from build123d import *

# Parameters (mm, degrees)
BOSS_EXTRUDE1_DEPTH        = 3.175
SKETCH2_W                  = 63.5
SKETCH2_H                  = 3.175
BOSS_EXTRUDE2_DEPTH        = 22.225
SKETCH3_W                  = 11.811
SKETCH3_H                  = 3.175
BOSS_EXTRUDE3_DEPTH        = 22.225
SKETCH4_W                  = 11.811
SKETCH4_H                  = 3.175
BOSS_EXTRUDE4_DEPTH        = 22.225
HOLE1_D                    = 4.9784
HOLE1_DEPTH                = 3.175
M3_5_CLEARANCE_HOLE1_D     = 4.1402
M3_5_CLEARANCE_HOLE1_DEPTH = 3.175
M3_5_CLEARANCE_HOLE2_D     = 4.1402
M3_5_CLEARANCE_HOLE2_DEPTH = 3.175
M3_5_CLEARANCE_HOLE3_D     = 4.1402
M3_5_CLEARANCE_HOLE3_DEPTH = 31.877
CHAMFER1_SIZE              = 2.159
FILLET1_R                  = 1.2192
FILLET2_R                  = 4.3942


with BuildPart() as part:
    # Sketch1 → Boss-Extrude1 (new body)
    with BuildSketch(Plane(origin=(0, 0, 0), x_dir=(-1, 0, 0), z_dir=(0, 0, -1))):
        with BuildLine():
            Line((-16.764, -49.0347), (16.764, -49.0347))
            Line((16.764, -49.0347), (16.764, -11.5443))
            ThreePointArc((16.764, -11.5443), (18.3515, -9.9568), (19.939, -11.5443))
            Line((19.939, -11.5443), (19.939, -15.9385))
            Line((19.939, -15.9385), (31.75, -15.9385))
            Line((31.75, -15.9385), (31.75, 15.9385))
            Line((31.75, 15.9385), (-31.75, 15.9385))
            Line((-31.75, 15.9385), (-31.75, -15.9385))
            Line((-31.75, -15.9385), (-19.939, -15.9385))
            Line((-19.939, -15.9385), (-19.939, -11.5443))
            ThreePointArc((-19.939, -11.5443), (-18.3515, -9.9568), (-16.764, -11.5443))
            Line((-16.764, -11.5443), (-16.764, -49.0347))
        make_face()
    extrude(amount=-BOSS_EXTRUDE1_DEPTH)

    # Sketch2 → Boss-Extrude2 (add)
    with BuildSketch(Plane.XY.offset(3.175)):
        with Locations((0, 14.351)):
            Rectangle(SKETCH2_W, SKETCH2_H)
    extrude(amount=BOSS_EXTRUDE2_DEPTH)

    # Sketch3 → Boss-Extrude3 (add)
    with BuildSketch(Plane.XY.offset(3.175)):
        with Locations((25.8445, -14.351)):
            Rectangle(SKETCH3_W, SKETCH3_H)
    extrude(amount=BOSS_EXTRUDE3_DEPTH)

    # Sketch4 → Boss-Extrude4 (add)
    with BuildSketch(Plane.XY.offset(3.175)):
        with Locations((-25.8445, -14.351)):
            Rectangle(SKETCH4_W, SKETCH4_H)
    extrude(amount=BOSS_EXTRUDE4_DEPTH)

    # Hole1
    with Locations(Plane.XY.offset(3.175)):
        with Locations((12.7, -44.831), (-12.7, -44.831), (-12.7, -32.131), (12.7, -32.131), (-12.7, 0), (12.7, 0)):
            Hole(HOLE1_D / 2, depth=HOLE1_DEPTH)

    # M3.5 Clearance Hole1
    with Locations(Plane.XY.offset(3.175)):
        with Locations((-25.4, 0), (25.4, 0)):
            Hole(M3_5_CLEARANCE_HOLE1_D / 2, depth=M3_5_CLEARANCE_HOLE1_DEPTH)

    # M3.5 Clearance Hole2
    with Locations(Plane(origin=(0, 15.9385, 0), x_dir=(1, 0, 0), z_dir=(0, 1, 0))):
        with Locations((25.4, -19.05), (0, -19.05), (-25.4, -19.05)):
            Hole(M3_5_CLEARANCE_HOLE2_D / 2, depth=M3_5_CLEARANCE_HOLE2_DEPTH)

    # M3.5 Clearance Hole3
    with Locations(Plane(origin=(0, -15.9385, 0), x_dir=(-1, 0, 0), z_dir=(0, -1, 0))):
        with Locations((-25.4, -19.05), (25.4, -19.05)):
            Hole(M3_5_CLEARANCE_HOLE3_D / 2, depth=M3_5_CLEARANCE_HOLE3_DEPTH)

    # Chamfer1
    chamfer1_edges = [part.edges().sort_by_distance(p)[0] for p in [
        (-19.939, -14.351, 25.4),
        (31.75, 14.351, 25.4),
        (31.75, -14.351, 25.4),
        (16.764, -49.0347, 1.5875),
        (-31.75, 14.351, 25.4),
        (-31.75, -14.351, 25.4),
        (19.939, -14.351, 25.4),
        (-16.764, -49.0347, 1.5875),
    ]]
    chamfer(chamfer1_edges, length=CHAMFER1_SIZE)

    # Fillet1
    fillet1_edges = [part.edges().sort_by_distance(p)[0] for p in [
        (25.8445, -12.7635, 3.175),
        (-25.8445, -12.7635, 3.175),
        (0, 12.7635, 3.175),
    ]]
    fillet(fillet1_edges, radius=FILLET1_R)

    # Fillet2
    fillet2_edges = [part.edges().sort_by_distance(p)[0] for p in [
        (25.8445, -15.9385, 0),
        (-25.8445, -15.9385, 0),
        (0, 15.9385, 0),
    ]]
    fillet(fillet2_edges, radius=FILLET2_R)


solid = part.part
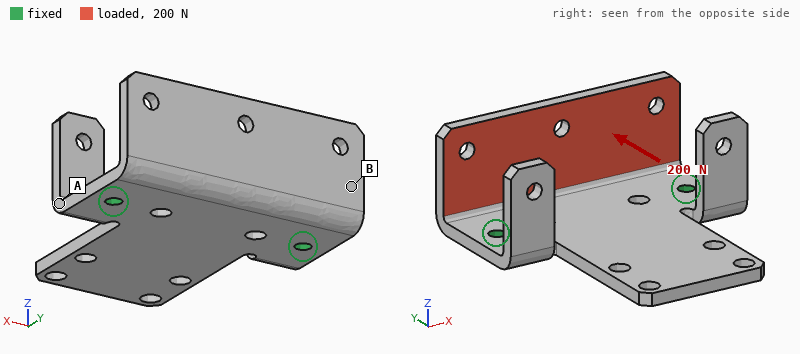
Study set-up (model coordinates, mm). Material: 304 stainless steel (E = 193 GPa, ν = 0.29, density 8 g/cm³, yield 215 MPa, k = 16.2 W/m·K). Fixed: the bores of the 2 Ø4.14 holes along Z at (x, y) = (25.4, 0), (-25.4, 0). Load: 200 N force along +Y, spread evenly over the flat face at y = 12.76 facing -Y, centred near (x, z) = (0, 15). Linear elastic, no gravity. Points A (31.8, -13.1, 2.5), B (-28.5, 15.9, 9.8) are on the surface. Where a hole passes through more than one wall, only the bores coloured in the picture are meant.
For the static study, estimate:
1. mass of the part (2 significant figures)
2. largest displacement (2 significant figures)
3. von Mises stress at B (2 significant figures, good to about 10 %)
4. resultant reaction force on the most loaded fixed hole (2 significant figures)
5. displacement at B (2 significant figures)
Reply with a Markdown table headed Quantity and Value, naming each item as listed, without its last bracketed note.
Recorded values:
| Quantity | Value |
|---|---|
| mass of the part | 120 g |
| largest displacement | 42 µm |
| von Mises stress at B | 10 MPa |
| resultant reaction force on the most loaded fixed hole | 100 N |
| displacement at B | 18 µm |
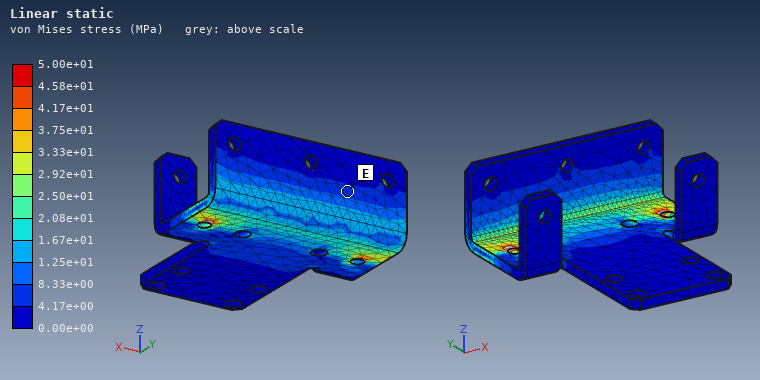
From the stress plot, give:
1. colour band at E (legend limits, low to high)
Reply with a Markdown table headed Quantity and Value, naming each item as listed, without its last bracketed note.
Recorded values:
| Quantity | Value |
|---|---|
| colour band at E | 4.17e+00 to 8.33e+00 MPa |
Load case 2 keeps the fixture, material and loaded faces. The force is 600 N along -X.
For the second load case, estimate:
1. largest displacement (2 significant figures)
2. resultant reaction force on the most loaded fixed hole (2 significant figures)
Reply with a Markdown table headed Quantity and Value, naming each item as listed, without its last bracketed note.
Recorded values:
| Quantity | Value |
|---|---|
| largest displacement | 24 µm |
| resultant reaction force on the most loaded fixed hole | 370 N |
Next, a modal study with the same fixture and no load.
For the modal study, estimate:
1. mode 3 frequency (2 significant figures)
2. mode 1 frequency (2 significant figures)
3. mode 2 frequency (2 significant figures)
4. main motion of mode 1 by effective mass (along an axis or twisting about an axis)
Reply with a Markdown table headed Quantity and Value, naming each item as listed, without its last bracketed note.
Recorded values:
| Quantity | Value |
|---|---|
| mode 3 frequency | 2700 Hz |
| mode 1 frequency | 990 Hz |
| mode 2 frequency | 2200 Hz |
| main motion of mode 1 by effective mass | along Z |
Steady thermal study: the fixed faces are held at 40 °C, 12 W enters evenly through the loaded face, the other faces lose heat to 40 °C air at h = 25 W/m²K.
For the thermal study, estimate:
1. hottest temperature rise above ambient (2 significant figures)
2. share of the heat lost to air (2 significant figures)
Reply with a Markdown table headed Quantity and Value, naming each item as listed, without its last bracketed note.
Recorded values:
| Quantity | Value |
|---|---|
| hottest temperature rise above ambient | 81 K |
| share of the heat lost to air | 50 % |
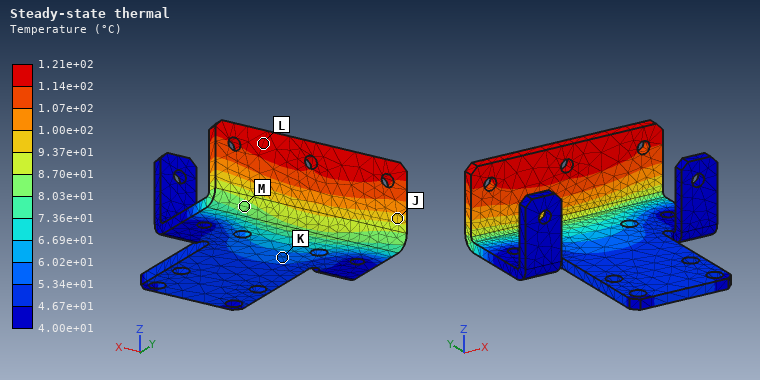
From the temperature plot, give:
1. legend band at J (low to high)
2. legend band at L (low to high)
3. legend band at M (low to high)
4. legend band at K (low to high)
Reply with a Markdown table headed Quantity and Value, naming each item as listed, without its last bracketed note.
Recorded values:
| Quantity | Value |
|---|---|
| legend band at J | 9.37e+01 to 1.00e+02 °C |
| legend band at L | 1.14e+02 to 1.21e+02 °C |
| legend band at M | 8.03e+01 to 8.70e+01 °C |
| legend band at K | 5.34e+01 to 6.02e+01 °C |
